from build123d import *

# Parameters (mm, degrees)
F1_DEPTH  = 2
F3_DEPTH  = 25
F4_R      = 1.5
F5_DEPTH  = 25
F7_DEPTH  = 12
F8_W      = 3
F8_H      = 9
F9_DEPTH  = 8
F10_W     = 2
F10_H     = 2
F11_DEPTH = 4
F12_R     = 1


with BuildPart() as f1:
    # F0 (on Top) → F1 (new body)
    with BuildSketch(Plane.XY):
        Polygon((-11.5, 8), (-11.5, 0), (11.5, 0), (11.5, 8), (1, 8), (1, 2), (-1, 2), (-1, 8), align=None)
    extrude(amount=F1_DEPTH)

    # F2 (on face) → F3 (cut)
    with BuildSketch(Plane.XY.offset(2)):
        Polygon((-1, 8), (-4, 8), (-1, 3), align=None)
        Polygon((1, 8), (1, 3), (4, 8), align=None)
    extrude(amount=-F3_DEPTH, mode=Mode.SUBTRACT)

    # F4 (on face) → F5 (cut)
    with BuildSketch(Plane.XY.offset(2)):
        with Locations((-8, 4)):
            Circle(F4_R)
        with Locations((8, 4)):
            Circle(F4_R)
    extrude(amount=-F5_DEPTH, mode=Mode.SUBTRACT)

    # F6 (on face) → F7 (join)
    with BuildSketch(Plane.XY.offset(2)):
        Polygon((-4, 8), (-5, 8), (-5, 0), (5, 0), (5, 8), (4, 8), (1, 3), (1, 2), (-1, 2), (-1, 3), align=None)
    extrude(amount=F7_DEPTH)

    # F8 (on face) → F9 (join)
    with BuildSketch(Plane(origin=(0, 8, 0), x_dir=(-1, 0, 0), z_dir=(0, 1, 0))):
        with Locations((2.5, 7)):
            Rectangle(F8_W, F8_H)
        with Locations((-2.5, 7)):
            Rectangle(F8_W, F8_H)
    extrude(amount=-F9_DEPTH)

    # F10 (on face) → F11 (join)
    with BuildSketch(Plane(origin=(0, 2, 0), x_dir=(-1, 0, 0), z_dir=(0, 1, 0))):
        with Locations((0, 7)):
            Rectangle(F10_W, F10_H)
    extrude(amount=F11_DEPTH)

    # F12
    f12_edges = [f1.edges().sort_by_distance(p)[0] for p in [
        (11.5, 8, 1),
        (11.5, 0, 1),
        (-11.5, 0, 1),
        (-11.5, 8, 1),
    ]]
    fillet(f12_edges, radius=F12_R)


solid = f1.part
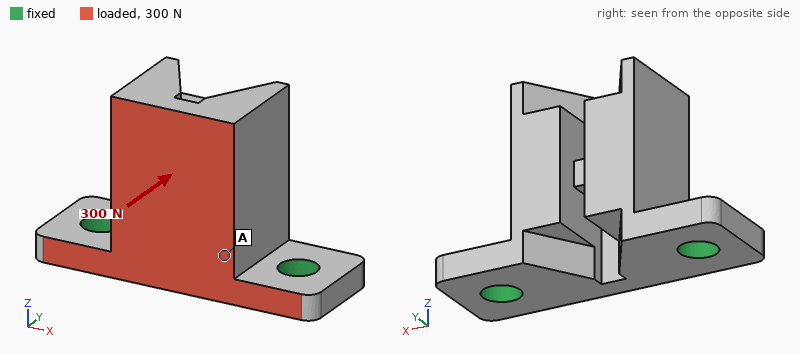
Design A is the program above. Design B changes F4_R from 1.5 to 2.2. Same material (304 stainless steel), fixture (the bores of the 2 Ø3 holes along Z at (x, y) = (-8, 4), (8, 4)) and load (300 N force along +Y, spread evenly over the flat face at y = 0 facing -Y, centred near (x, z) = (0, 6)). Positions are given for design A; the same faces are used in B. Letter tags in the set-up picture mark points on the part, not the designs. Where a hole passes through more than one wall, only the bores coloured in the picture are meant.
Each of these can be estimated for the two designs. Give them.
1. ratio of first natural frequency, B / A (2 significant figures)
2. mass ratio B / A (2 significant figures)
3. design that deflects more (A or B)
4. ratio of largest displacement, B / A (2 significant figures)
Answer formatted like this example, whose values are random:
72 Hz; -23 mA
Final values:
1.3; 0.97; A; 0.64
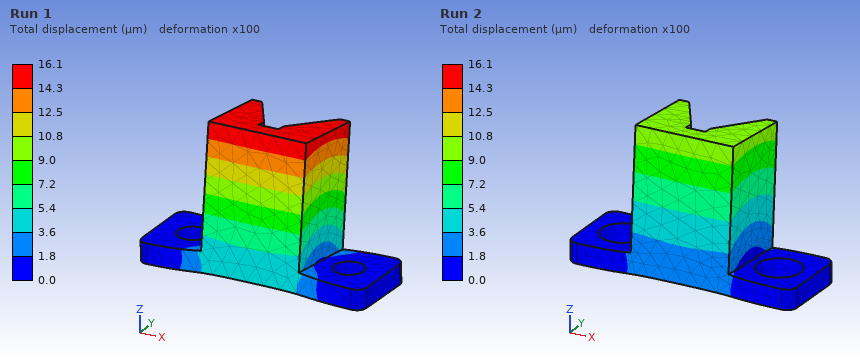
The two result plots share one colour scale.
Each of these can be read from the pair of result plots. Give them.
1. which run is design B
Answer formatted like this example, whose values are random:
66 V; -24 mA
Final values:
Run 2
